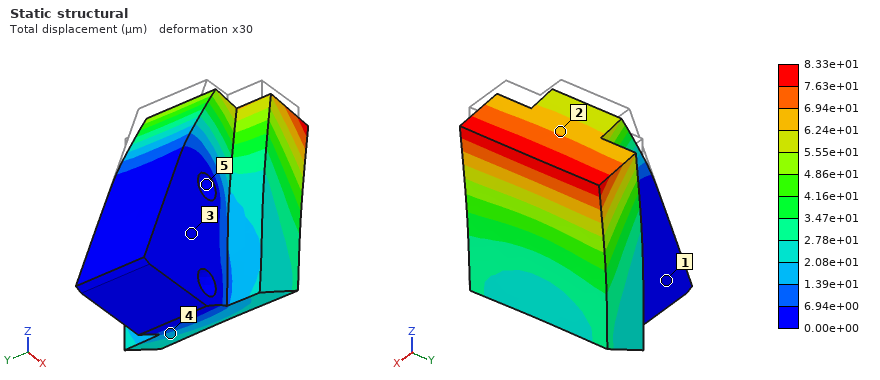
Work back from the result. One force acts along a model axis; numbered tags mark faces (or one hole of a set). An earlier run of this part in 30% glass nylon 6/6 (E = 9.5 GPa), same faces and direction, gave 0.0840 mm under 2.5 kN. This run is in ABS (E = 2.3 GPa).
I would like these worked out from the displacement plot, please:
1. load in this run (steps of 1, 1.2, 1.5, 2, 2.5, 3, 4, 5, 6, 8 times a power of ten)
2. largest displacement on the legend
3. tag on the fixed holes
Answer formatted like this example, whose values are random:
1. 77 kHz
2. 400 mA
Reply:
1. 600 N
2. 8.33e+01 µm
3. 5
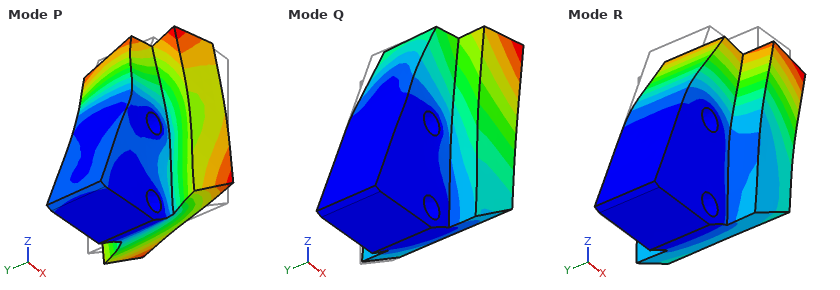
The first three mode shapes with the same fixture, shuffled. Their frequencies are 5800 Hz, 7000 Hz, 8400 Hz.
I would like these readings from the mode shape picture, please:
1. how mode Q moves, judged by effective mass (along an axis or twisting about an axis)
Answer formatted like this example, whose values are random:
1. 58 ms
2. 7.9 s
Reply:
1. along Y
